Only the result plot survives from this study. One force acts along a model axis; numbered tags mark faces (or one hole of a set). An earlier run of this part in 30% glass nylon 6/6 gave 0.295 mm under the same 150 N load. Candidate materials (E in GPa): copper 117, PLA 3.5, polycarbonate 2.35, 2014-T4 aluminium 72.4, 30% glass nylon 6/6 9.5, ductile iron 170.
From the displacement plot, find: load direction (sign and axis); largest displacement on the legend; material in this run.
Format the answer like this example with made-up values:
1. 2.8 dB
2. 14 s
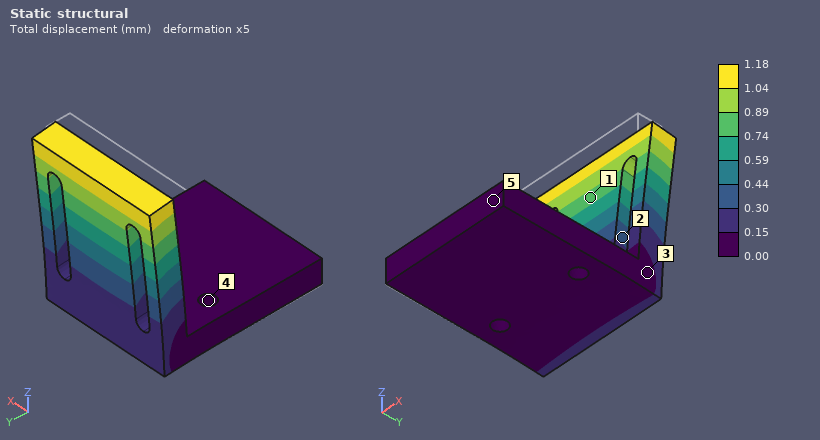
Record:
1. +Y
2. 1.18 mm
3. polycarbonate
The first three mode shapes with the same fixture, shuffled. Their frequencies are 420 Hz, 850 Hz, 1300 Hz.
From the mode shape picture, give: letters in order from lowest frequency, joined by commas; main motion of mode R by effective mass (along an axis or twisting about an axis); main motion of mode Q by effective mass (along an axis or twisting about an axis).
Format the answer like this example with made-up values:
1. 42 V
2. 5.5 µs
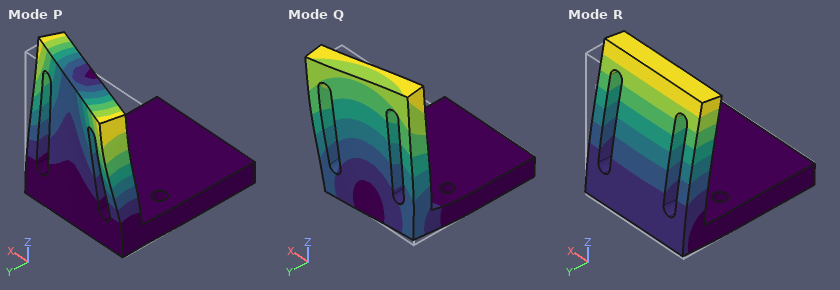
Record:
1. R, Q, P
2. along Y
3. along X
